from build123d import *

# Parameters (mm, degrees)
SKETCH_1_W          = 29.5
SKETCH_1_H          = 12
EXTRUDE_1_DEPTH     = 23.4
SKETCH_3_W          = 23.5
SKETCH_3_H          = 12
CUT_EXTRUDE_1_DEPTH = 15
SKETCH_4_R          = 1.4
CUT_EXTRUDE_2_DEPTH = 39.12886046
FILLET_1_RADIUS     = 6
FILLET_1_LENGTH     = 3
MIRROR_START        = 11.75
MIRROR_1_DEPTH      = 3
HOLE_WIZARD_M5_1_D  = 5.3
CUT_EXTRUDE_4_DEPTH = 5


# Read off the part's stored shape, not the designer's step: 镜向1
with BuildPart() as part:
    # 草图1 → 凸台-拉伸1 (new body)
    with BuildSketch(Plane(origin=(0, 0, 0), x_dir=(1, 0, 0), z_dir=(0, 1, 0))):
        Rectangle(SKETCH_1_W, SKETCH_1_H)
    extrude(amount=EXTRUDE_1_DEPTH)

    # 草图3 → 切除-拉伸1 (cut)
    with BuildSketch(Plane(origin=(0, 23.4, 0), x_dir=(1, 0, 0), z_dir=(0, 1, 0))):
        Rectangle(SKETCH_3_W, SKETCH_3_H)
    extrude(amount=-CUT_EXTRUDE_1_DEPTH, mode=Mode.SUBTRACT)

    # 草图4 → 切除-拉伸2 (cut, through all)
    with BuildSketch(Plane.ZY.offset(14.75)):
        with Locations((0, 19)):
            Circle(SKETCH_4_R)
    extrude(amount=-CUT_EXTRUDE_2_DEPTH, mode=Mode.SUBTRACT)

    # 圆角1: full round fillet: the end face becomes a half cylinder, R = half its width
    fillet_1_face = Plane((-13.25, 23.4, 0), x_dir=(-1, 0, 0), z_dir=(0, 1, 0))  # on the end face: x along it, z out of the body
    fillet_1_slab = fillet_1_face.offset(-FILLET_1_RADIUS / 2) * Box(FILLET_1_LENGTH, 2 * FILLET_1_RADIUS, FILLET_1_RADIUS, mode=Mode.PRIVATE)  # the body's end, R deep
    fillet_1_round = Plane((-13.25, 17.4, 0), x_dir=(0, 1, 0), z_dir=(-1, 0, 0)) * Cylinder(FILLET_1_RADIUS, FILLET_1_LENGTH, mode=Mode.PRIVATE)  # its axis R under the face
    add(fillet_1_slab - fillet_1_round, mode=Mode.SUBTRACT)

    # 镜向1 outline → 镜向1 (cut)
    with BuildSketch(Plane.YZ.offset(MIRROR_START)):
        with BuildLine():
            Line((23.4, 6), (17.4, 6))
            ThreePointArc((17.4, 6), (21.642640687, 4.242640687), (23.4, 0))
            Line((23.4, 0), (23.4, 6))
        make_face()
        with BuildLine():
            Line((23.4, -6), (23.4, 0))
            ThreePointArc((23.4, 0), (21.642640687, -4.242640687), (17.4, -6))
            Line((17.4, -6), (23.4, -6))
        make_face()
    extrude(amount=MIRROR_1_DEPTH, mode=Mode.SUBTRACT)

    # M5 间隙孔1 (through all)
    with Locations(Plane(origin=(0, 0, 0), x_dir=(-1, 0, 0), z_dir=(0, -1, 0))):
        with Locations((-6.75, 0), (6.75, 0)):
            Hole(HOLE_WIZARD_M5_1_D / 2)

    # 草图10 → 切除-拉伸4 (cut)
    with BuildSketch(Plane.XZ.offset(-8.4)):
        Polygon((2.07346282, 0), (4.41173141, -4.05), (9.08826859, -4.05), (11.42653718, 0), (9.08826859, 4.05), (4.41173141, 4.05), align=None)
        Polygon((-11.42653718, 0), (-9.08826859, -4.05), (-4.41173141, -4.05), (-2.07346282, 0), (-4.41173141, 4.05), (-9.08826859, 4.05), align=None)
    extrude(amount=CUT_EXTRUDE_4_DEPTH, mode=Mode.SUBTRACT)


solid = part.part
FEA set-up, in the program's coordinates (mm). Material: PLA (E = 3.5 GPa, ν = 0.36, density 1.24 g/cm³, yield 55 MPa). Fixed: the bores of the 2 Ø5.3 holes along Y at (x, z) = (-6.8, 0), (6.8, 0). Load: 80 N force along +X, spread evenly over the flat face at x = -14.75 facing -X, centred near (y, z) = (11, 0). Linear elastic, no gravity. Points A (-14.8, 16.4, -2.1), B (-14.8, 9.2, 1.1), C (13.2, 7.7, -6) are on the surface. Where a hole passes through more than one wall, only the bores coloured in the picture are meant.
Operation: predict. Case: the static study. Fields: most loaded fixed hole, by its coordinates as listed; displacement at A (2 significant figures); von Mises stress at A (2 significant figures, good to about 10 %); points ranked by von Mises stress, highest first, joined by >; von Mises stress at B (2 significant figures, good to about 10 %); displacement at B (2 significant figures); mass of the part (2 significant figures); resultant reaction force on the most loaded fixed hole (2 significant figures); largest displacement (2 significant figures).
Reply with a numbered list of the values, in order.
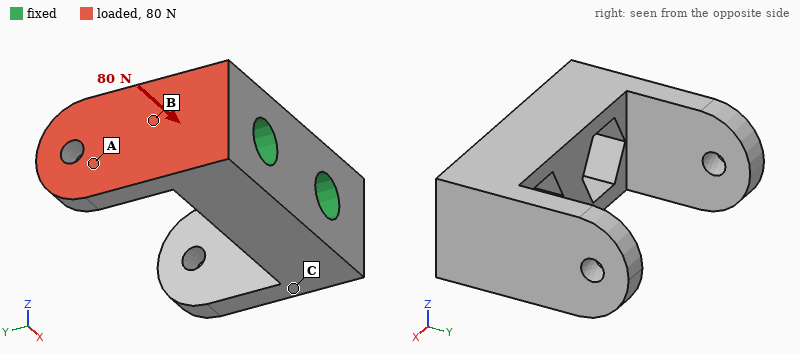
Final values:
1. (6.8, 0)
2. 0.21 mm
3. 4.2 MPa
4. B > A > C
5. 14 MPa
6. 0.066 mm
7. 4.0 g
8. 57 N
9. 0.40 mm
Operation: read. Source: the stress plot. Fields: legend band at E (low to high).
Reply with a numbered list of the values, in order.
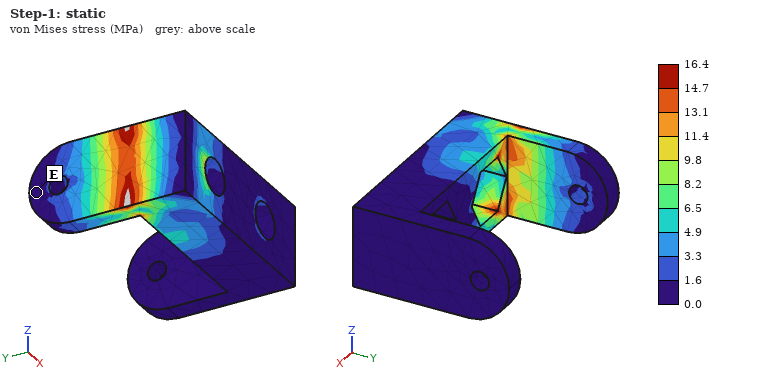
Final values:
1. 0.0 to 1.6 MPa
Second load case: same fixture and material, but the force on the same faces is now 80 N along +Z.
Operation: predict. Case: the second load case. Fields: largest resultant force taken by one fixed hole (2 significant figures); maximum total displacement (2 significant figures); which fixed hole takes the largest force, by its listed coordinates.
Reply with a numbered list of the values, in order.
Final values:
1. 91 N
2. 0.15 mm
3. (-6.8, 0)
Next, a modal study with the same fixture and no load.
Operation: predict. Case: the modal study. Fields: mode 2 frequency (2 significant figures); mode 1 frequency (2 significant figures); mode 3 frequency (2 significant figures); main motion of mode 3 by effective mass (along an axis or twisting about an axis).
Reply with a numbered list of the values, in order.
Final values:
1. 3000 Hz
2. 3000 Hz
3. 4300 Hz
4. along Z
